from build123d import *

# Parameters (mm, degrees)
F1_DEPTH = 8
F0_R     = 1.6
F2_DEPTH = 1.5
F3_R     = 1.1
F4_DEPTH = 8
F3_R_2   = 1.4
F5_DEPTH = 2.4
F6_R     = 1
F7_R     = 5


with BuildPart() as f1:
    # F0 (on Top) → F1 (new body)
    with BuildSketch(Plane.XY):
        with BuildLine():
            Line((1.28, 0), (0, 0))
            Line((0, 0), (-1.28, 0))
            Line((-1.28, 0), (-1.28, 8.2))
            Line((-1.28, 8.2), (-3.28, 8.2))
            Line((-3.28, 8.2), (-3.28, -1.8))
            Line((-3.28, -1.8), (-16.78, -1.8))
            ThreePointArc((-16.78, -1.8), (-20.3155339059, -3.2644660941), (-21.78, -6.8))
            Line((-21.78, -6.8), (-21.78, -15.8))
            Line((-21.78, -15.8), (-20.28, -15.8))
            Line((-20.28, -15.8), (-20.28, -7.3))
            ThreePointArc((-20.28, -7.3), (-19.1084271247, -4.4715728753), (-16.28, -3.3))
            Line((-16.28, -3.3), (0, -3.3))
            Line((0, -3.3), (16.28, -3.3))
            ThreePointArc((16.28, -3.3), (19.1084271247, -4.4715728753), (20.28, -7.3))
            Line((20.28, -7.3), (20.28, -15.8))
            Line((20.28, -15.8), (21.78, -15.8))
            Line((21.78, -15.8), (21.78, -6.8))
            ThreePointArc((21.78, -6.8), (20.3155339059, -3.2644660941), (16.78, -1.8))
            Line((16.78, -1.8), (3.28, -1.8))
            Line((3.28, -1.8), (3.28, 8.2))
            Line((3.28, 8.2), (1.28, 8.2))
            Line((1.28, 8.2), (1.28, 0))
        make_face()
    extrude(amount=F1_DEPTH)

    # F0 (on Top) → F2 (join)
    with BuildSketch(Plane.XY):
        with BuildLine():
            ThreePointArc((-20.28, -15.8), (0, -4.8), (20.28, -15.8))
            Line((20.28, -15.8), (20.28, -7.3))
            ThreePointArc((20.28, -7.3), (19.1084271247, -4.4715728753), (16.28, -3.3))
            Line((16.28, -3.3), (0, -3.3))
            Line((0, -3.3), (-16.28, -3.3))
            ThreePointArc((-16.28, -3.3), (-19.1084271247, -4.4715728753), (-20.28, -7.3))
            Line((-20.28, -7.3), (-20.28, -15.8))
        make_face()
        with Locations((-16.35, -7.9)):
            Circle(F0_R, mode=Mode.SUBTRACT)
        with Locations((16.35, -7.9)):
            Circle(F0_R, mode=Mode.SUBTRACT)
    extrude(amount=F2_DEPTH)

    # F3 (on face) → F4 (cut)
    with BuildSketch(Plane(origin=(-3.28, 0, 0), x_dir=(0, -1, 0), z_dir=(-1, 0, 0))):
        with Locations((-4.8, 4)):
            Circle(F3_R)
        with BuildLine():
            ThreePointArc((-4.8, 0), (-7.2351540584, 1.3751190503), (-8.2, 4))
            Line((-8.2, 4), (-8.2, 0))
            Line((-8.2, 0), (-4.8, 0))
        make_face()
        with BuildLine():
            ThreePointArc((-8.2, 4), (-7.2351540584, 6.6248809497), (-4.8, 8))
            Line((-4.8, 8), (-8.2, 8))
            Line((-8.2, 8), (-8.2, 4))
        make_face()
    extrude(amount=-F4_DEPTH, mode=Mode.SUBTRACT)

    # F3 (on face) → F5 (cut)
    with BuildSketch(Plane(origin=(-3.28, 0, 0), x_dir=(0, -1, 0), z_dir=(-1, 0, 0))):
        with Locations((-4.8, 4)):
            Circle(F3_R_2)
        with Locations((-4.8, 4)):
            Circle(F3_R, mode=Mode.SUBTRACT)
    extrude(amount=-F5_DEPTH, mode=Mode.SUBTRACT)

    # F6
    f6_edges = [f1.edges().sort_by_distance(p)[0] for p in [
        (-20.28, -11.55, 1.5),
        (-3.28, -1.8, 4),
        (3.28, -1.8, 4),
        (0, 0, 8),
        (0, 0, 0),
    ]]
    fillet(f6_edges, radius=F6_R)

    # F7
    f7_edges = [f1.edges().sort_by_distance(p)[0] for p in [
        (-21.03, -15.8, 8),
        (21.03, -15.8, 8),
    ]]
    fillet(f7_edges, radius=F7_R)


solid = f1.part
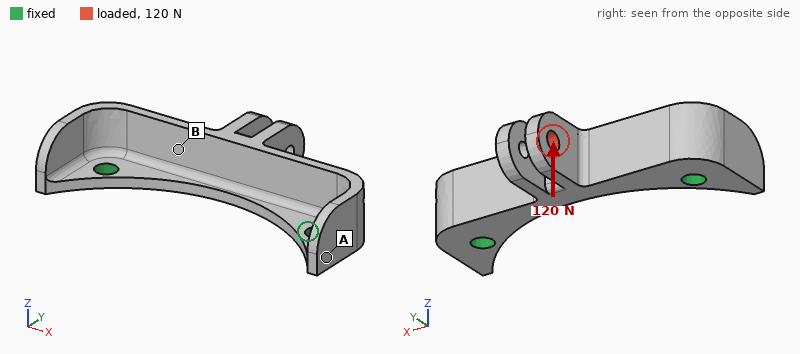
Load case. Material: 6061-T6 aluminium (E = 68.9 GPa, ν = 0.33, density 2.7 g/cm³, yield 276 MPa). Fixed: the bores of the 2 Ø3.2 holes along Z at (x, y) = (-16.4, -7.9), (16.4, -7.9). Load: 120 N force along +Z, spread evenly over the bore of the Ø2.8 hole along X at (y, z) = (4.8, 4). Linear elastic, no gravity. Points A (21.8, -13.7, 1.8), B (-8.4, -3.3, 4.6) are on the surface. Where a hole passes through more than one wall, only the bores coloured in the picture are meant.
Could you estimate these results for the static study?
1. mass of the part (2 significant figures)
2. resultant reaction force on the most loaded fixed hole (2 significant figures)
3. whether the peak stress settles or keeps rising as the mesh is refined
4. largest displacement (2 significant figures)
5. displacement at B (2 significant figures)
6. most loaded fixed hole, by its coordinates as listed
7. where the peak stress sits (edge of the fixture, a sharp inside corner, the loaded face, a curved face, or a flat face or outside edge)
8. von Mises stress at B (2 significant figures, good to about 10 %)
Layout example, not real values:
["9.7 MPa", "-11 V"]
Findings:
["3.7 g", "89 N", "keeps rising", "0.25 mm", "0.057 mm", "(-16.4, -7.9)", "edge of the fixture", "60 MPa"]
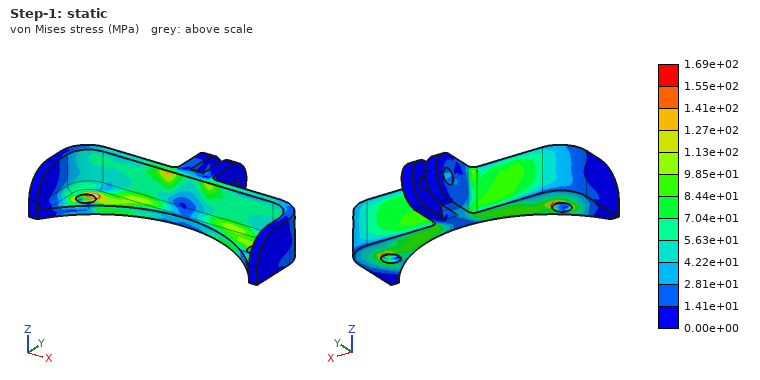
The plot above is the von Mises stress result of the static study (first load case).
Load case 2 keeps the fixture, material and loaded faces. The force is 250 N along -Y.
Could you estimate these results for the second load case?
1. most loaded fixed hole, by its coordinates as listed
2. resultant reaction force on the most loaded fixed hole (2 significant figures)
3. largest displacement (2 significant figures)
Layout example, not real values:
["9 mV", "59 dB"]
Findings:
["(-16.4, -7.9)", "220 N", "0.18 mm"]
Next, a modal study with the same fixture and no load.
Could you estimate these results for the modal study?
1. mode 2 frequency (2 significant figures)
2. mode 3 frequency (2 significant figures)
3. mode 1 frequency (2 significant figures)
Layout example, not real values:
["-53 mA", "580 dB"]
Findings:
["14 kHz", "14 kHz", "4600 Hz"]
